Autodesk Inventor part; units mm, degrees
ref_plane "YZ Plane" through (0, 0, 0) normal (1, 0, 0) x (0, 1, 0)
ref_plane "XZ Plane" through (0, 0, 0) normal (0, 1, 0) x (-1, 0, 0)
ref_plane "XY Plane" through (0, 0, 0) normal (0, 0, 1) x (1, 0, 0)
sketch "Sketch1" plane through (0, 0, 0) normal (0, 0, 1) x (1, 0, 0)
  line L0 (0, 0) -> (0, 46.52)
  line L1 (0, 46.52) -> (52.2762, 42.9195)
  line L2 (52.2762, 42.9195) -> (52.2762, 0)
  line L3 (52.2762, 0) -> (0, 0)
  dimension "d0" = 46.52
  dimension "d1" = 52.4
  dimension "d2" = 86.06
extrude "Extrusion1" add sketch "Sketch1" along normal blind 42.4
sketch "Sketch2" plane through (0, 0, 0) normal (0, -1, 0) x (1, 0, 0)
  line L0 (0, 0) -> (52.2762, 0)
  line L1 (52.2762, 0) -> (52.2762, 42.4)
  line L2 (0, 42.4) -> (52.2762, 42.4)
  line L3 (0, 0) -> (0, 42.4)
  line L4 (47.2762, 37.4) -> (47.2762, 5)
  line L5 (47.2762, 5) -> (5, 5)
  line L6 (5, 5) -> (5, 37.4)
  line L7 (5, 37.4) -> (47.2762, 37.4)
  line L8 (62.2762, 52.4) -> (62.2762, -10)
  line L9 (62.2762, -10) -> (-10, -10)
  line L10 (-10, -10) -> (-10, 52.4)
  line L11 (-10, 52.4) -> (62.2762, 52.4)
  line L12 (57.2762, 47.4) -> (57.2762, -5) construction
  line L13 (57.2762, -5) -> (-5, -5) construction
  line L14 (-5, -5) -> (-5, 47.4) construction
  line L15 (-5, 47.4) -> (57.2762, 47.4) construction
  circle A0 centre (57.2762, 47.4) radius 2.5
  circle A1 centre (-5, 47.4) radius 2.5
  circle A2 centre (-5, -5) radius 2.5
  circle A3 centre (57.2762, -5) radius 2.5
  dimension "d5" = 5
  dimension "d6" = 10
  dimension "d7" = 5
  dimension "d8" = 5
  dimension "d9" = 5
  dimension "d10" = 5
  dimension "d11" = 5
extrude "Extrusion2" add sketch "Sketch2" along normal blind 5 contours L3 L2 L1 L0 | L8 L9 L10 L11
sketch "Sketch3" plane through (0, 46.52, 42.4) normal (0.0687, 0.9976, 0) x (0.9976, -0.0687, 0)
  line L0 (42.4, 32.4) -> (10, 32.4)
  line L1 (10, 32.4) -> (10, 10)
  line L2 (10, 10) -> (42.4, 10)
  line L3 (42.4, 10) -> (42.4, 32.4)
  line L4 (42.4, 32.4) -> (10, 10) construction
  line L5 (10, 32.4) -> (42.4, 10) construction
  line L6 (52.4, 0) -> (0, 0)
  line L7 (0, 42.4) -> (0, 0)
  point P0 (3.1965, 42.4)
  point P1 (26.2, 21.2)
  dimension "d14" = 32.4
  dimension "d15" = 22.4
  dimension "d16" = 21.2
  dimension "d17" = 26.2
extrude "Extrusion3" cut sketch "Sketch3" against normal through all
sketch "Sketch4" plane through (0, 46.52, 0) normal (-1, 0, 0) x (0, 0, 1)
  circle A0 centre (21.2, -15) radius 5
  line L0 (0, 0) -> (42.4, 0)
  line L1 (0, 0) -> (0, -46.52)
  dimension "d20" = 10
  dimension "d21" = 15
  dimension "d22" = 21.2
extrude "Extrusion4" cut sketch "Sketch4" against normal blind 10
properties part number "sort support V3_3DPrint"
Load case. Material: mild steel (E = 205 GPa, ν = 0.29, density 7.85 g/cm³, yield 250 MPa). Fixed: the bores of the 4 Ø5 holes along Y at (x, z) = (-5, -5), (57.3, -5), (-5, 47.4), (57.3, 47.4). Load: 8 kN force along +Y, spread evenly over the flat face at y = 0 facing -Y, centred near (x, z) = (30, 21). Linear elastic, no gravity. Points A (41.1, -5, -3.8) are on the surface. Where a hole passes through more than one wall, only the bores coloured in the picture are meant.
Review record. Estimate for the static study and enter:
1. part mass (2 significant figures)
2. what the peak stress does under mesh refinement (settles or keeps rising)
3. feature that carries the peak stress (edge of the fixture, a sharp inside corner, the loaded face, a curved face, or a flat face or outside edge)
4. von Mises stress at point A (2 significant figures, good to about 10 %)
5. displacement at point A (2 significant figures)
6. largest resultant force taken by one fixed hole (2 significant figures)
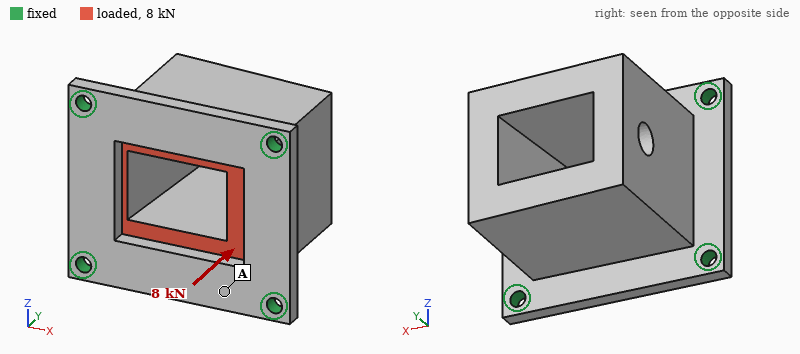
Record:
640 g
keeps rising
edge of the fixture
32 MPa
11 µm
2.6 kN
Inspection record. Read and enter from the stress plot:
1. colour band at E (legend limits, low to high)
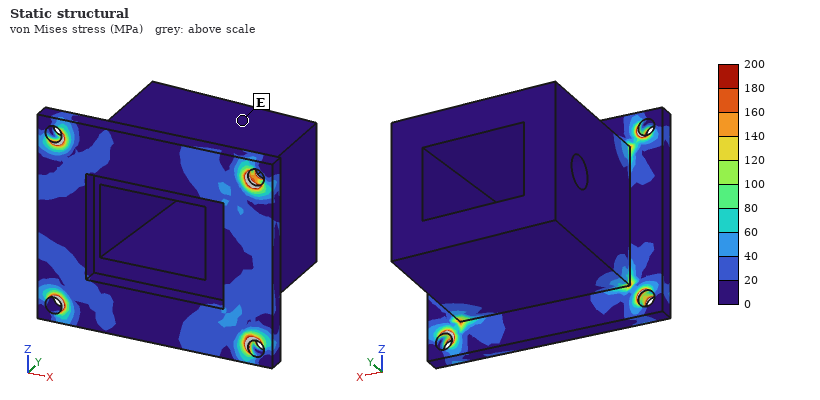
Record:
0 to 20 MPa
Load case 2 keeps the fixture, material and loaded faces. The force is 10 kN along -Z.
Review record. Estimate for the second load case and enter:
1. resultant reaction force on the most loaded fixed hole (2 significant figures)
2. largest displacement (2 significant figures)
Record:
3.3 kN
8.0 µm
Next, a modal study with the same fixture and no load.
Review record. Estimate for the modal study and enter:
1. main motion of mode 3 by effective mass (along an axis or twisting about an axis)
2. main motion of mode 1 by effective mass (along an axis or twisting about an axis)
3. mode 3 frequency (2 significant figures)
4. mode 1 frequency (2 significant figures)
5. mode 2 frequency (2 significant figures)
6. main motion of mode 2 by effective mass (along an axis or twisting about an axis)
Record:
along Y
along Z
5300 Hz
3900 Hz
4500 Hz
along X
